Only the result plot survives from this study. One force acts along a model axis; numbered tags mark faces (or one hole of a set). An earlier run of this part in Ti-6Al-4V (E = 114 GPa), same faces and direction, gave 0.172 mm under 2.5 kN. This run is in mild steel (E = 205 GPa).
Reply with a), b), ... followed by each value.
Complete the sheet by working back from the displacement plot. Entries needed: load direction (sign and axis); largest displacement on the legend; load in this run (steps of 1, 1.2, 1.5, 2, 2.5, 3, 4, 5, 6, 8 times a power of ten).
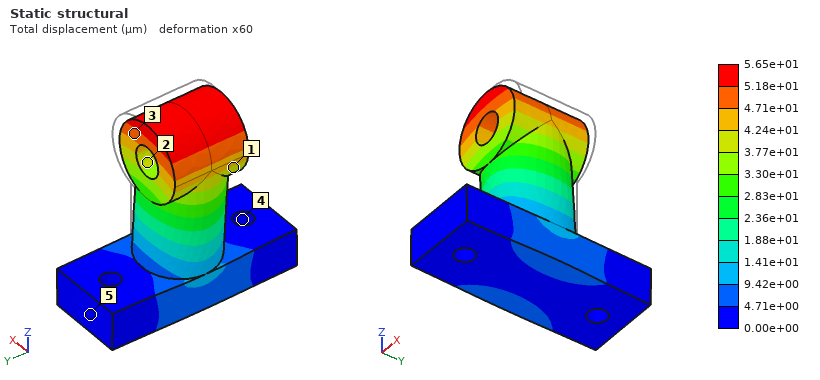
a) -X
b) 5.65e+01 µm
c) 1.5 kN
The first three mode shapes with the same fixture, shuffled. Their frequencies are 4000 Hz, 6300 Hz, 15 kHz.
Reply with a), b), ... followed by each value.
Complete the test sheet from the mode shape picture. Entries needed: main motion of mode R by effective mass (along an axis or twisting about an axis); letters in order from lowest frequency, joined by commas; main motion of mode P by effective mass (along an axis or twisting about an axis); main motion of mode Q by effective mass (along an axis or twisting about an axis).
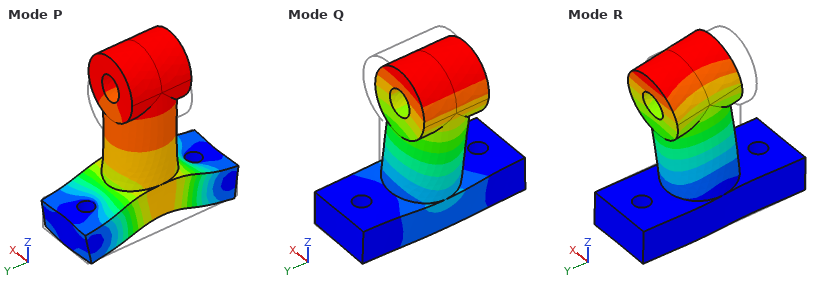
a) along Y
b) Q, R, P
c) along Z
d) along X
